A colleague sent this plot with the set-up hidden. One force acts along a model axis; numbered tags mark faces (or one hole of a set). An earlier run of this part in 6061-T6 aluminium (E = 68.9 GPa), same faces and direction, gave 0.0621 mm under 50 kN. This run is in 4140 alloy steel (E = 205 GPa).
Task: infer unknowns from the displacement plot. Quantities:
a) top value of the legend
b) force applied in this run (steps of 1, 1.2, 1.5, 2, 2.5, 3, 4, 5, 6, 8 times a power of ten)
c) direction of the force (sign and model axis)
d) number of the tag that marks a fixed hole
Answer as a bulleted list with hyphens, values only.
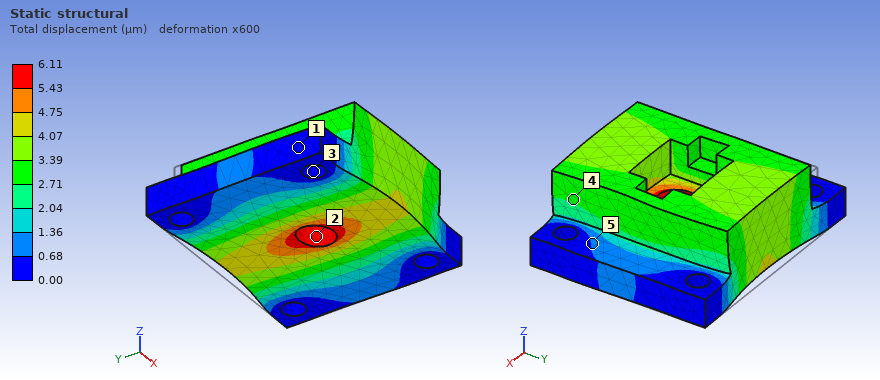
- 6.11 µm
- 15 kN
- -Y
- 3
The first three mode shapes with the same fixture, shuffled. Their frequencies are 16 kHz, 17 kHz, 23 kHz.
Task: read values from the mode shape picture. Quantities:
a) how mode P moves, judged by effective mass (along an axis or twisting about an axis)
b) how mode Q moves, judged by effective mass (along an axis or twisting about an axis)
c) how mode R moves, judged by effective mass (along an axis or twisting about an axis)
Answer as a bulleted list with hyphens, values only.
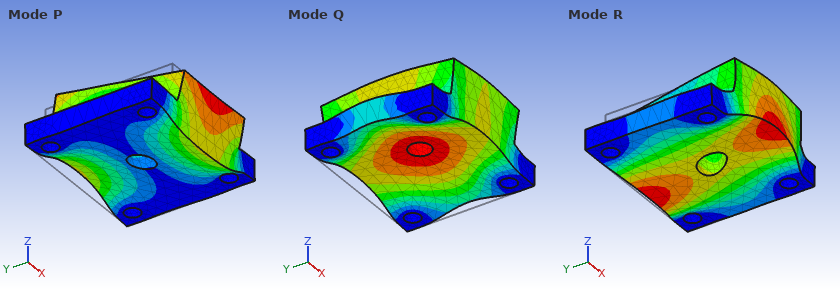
- along Y
- along Z
- along Y
